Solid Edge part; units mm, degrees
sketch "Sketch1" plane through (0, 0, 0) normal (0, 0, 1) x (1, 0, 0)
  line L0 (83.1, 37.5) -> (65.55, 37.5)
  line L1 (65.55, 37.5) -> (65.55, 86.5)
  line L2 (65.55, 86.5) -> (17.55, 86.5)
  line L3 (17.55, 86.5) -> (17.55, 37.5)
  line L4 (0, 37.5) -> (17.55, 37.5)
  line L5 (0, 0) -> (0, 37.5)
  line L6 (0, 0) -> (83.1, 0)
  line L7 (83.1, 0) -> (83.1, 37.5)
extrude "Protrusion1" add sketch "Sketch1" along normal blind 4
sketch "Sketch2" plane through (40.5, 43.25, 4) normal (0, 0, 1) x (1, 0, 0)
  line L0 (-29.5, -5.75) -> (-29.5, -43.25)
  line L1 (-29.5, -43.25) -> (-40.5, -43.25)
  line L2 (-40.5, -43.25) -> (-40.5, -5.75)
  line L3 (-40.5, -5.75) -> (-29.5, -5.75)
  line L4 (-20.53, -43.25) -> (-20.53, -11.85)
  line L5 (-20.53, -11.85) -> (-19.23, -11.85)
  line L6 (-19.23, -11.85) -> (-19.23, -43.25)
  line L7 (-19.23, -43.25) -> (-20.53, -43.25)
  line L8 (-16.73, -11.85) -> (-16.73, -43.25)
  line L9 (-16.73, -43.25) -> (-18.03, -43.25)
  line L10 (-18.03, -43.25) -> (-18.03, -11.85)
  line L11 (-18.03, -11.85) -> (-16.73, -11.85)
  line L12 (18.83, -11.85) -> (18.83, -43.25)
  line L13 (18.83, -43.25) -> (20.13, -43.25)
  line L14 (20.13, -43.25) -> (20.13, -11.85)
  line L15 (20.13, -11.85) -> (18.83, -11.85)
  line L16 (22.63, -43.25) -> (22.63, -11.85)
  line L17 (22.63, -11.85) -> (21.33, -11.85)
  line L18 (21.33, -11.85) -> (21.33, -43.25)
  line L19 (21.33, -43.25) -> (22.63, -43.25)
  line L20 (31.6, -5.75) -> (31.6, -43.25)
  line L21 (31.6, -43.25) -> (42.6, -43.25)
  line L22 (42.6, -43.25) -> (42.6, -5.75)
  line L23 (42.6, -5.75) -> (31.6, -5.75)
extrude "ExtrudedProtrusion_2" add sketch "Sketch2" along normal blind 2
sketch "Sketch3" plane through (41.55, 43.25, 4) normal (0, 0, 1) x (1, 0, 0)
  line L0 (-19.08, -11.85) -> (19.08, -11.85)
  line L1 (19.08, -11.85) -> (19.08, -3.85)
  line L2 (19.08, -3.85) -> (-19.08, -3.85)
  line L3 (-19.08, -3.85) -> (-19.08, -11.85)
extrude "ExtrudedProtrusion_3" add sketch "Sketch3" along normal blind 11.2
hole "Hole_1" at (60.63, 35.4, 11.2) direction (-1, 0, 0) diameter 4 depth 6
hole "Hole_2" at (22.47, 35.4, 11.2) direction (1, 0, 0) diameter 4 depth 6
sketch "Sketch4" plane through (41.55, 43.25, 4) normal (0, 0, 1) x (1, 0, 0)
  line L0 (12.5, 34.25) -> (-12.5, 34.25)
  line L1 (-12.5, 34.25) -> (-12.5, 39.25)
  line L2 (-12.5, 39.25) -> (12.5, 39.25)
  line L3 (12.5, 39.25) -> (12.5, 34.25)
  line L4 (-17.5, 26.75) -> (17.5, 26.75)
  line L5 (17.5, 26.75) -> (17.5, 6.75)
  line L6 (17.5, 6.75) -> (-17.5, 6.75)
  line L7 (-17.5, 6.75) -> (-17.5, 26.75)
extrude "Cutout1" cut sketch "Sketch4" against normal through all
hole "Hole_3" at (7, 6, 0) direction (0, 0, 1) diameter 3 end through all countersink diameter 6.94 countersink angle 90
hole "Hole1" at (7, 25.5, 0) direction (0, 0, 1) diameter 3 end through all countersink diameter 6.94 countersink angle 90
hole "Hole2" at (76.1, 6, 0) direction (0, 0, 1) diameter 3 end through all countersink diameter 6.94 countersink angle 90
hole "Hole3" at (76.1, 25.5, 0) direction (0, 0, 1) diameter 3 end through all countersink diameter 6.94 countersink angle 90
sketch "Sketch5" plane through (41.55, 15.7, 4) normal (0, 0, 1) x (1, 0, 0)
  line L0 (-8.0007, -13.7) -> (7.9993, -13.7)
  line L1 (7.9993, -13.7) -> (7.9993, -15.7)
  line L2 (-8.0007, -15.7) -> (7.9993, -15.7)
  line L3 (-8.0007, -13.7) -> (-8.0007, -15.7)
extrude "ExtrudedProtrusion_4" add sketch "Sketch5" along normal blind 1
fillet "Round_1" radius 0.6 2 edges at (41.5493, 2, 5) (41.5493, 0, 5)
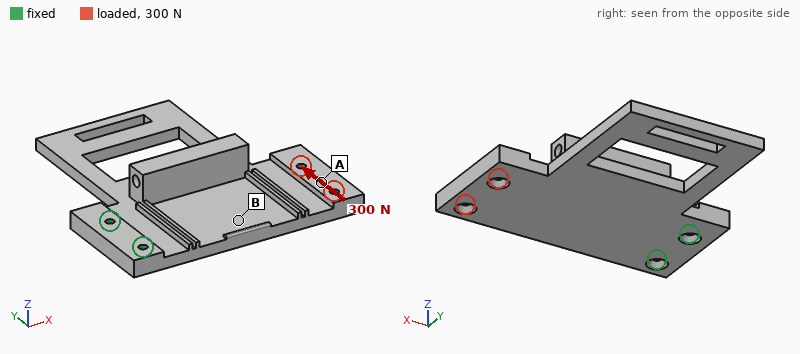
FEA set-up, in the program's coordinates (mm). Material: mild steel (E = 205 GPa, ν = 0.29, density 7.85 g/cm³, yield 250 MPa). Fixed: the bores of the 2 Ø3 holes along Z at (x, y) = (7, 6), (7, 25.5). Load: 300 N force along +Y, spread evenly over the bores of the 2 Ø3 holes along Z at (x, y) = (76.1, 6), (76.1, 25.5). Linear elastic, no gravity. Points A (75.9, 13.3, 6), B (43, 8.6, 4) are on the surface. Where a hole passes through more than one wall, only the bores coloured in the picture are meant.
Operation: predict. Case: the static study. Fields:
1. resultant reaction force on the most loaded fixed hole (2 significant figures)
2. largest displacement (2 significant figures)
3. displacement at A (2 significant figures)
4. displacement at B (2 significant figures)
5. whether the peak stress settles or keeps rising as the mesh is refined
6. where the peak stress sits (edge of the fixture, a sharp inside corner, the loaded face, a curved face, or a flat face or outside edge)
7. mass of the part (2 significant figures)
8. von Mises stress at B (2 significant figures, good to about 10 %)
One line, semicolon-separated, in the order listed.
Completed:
990 N; 30 µm; 16 µm; 7.4 µm; keeps rising; edge of the fixture; 190 g; 8.6 MPa
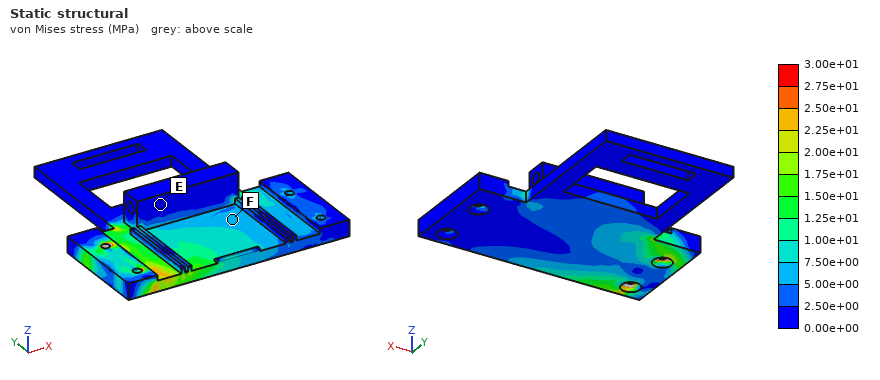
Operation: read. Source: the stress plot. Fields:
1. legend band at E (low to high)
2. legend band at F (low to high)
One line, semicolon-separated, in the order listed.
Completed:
0.00e+00 to 2.50e+00 MPa; 5.00e+00 to 7.50e+00 MPa
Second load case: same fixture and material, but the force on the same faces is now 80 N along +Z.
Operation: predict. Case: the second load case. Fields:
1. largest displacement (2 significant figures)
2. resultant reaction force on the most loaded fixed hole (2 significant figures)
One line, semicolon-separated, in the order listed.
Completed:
0.18 mm; 62 N
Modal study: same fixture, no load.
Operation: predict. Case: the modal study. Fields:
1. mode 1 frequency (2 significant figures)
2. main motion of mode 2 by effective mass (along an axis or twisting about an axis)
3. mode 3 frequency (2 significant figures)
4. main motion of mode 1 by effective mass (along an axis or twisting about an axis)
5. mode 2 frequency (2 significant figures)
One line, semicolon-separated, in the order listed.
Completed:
460 Hz; twisting about X; 2200 Hz; along Z; 800 Hz
